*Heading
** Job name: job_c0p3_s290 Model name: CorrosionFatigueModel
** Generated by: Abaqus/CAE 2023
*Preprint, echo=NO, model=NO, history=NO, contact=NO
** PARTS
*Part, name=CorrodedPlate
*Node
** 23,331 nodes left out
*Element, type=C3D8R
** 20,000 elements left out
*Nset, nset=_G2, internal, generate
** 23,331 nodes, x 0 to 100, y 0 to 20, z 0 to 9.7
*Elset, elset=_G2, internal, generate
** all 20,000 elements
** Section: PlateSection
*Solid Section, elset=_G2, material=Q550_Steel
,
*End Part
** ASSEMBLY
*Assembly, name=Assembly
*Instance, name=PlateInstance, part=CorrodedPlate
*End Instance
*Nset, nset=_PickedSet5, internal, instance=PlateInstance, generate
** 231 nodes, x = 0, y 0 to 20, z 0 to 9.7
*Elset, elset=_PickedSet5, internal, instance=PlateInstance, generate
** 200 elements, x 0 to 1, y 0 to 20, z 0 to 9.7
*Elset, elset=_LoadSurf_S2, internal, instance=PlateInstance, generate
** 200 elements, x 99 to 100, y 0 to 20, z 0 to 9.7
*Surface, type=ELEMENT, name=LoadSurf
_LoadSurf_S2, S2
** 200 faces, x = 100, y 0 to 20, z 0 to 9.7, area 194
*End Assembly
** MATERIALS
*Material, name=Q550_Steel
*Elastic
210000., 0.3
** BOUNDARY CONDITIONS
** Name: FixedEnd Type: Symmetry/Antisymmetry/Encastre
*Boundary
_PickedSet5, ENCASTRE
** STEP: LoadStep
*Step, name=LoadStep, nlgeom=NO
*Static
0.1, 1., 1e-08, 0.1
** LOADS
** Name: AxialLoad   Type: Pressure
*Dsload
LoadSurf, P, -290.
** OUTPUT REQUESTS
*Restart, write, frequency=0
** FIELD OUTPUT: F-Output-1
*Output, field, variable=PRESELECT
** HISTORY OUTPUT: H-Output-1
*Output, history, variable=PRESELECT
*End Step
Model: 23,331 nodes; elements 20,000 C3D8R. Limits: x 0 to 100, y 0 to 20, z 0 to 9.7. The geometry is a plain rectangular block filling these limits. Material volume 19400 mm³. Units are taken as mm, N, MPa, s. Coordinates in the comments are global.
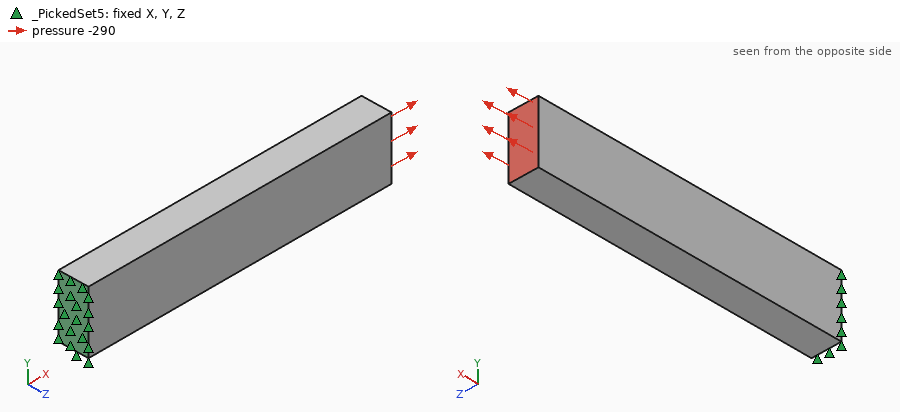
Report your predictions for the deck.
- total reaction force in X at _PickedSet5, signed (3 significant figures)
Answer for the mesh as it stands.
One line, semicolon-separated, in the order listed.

-56300 N
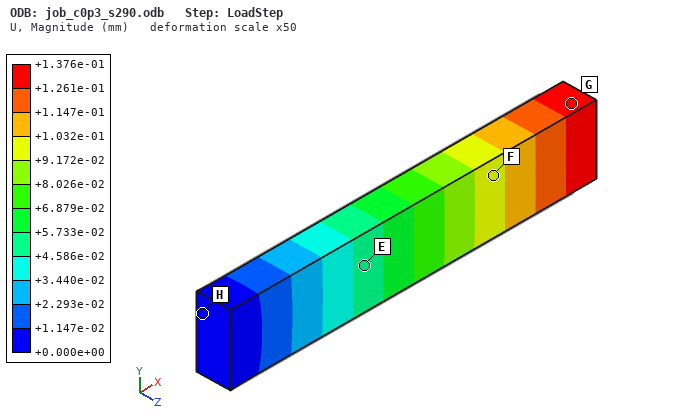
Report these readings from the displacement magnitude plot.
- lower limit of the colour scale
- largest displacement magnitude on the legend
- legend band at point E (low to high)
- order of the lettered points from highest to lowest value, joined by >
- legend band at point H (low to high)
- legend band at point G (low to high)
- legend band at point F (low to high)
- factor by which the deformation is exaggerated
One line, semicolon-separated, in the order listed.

+0.000e+00 mm; +1.376e-01 mm; +4.586e-02 to +5.733e-02 mm; G > F > E > H; +0.000e+00 to +1.147e-02 mm; +1.261e-01 to +1.376e-01 mm; +9.172e-02 to +1.032e-01 mm; 50
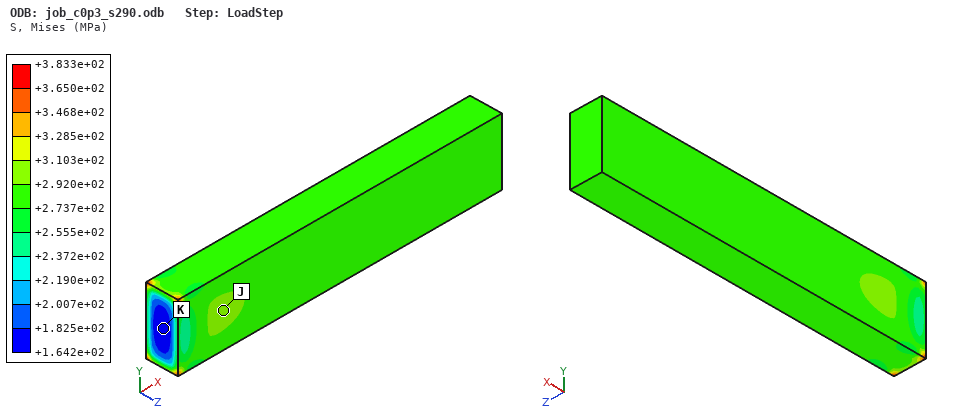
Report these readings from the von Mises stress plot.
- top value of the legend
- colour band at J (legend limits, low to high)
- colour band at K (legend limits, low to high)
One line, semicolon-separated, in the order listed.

+3.833e+02 MPa; +2.920e+02 to +3.103e+02 MPa; +1.642e+02 to +1.825e+02 MPa
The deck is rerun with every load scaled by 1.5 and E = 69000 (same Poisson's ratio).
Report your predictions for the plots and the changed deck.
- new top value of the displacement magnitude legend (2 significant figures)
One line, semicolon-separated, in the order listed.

0.63 mm
